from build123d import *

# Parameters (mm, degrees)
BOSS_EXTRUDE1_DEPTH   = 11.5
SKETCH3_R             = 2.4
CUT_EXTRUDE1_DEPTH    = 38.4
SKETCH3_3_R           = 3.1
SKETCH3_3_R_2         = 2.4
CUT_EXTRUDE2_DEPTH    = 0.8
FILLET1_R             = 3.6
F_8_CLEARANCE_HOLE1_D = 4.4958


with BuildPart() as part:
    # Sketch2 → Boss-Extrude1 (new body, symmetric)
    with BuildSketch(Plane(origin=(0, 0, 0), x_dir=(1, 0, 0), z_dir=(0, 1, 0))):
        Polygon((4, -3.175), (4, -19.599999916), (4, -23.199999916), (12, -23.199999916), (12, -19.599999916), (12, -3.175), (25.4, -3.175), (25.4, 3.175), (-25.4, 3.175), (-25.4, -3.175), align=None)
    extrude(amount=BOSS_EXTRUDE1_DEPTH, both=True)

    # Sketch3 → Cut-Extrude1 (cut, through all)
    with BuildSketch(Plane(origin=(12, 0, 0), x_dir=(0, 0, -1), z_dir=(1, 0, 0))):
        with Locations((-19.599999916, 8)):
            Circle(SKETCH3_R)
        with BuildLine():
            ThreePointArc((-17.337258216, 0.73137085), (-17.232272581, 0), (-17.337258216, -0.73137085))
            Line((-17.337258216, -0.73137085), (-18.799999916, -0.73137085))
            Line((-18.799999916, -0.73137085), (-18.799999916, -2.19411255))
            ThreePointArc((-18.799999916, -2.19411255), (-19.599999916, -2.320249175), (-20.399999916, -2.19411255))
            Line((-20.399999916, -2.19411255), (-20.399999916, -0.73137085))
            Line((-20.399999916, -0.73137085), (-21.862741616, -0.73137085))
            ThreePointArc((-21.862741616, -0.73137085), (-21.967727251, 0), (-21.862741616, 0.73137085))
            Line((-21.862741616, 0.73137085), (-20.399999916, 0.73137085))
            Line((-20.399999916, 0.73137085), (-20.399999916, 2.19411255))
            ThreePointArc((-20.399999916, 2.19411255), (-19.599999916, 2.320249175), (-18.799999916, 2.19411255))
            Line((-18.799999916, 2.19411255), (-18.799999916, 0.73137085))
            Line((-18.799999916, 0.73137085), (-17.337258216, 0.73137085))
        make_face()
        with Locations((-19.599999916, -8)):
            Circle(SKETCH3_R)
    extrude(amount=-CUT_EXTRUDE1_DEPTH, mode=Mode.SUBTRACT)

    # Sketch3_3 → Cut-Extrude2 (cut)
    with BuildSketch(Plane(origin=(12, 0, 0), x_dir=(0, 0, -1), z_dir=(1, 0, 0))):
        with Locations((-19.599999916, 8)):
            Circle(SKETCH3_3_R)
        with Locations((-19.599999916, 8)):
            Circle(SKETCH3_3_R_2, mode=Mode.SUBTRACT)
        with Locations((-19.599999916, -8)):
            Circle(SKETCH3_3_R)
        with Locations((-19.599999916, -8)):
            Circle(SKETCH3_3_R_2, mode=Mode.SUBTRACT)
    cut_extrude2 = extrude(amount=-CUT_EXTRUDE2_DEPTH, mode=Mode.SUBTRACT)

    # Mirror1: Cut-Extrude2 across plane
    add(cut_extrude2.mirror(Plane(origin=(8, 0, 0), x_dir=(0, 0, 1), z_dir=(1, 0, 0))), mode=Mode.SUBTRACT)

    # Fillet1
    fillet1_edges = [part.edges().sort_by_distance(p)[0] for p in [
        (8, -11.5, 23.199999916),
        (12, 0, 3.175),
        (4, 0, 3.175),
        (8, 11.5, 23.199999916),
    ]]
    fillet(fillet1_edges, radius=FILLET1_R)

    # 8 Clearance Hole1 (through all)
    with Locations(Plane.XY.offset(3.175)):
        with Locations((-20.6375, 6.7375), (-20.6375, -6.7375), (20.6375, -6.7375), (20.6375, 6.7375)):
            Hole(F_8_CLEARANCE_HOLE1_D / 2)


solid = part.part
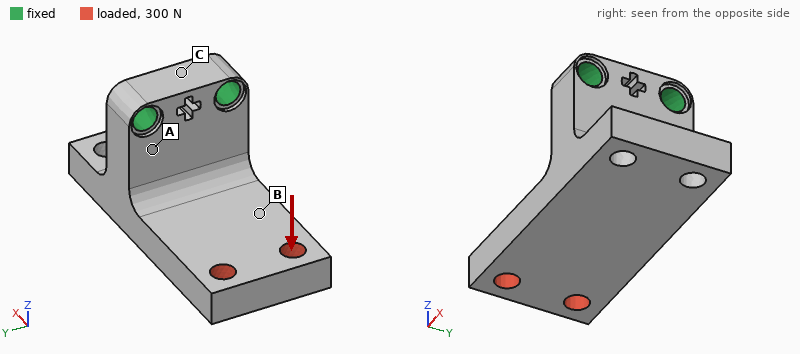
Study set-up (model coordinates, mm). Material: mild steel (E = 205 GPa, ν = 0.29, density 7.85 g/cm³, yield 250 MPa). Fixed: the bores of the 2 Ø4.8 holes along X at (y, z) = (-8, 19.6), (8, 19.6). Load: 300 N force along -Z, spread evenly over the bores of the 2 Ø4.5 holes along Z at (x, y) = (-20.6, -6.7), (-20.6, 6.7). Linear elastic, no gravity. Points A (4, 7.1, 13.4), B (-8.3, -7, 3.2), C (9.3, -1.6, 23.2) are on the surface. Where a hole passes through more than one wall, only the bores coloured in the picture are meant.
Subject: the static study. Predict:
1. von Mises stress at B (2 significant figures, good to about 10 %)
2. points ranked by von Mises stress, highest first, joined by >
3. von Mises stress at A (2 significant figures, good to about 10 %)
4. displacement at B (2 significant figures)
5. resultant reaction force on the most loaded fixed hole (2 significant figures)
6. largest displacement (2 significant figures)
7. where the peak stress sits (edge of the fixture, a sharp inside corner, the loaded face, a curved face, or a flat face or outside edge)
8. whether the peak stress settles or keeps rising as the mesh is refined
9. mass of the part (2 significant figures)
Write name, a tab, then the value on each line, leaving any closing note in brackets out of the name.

von Mises stress at B	24 MPa
points ranked by von Mises stress, highest first, joined by >	A > B > C
von Mises stress at A	38 MPa
displacement at B	18 µm
resultant reaction force on the most loaded fixed hole	160 N
largest displacement	49 µm
where the peak stress sits	edge of the fixture
whether the peak stress settles or keeps rising as the mesh is refined	keeps rising
mass of the part	81 g
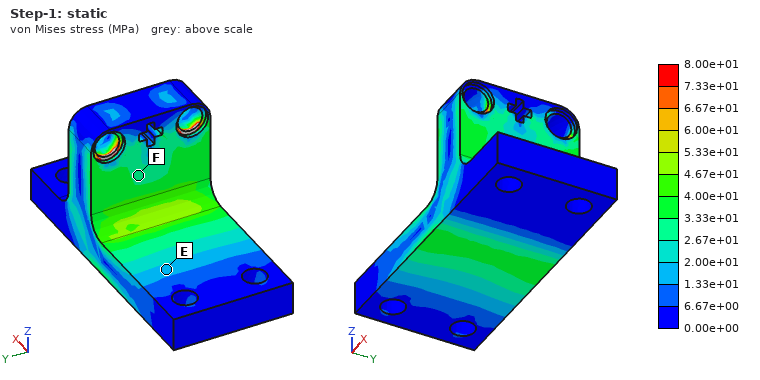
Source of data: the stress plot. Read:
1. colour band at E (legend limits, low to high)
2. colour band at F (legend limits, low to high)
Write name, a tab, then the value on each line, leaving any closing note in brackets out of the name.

colour band at E	1.33e+01 to 2.00e+01 MPa
colour band at F	2.67e+01 to 3.33e+01 MPa
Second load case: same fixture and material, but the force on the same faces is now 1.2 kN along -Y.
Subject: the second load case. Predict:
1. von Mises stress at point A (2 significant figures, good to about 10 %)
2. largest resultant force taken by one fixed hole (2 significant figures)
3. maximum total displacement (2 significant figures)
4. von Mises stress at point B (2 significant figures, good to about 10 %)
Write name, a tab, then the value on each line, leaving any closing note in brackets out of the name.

von Mises stress at point A	95 MPa
largest resultant force taken by one fixed hole	2.3 kN
maximum total displacement	67 µm
von Mises stress at point B	27 MPa
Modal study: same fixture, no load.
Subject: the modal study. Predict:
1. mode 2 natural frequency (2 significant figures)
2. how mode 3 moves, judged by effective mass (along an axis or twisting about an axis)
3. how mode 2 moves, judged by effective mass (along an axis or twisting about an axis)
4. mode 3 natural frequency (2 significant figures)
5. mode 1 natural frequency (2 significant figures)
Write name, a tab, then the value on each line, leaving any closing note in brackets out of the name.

mode 2 natural frequency	5400 Hz
how mode 3 moves, judged by effective mass	along X
how mode 2 moves, judged by effective mass	along Y
mode 3 natural frequency	8000 Hz
mode 1 natural frequency	3200 Hz
